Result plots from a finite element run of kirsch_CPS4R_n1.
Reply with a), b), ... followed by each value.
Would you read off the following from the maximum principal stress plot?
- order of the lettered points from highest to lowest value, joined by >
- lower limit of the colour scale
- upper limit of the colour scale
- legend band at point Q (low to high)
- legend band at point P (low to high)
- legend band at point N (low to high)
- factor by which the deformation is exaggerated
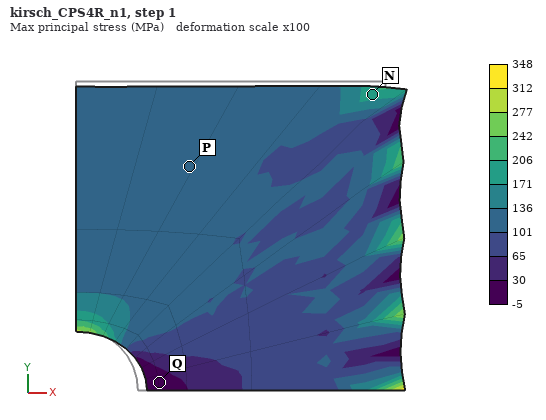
a) N > P > Q
b) -5 MPa
c) 348 MPa
d) -5 to 30 MPa
e) 101 to 136 MPa
f) 171 to 206 MPa
g) 100
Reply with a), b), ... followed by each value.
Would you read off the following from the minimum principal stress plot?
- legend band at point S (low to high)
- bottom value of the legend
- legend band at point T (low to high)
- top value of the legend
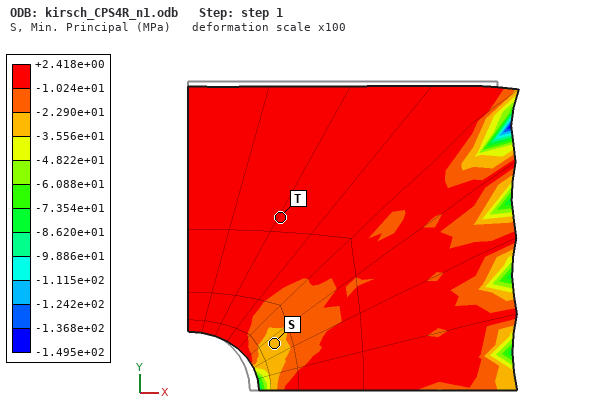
a) -3.556e+01 to -2.290e+01 MPa
b) -1.495e+02 MPa
c) -1.024e+01 to +2.418e+00 MPa
d) +2.418e+00 MPa
